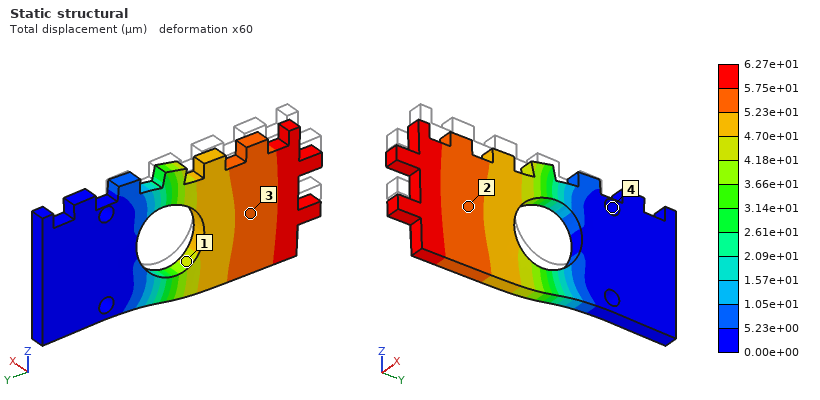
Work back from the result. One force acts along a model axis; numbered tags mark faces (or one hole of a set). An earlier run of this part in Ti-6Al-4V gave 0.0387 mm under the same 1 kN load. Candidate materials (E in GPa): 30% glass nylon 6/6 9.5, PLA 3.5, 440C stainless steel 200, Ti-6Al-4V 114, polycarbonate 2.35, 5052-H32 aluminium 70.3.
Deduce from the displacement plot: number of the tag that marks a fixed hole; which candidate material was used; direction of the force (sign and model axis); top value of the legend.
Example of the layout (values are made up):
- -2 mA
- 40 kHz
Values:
- 4
- 5052-H32 aluminium
- -Z
- 6.27e+01 µm
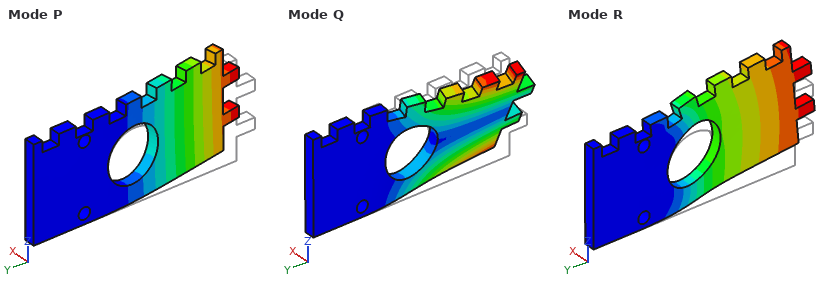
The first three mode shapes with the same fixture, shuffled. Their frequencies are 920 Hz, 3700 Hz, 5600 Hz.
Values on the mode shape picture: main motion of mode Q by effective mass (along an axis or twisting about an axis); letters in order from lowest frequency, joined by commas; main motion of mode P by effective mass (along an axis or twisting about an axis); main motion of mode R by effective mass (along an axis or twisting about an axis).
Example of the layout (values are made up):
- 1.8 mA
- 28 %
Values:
- twisting about Y
- P, Q, R
- along X
- along Z
